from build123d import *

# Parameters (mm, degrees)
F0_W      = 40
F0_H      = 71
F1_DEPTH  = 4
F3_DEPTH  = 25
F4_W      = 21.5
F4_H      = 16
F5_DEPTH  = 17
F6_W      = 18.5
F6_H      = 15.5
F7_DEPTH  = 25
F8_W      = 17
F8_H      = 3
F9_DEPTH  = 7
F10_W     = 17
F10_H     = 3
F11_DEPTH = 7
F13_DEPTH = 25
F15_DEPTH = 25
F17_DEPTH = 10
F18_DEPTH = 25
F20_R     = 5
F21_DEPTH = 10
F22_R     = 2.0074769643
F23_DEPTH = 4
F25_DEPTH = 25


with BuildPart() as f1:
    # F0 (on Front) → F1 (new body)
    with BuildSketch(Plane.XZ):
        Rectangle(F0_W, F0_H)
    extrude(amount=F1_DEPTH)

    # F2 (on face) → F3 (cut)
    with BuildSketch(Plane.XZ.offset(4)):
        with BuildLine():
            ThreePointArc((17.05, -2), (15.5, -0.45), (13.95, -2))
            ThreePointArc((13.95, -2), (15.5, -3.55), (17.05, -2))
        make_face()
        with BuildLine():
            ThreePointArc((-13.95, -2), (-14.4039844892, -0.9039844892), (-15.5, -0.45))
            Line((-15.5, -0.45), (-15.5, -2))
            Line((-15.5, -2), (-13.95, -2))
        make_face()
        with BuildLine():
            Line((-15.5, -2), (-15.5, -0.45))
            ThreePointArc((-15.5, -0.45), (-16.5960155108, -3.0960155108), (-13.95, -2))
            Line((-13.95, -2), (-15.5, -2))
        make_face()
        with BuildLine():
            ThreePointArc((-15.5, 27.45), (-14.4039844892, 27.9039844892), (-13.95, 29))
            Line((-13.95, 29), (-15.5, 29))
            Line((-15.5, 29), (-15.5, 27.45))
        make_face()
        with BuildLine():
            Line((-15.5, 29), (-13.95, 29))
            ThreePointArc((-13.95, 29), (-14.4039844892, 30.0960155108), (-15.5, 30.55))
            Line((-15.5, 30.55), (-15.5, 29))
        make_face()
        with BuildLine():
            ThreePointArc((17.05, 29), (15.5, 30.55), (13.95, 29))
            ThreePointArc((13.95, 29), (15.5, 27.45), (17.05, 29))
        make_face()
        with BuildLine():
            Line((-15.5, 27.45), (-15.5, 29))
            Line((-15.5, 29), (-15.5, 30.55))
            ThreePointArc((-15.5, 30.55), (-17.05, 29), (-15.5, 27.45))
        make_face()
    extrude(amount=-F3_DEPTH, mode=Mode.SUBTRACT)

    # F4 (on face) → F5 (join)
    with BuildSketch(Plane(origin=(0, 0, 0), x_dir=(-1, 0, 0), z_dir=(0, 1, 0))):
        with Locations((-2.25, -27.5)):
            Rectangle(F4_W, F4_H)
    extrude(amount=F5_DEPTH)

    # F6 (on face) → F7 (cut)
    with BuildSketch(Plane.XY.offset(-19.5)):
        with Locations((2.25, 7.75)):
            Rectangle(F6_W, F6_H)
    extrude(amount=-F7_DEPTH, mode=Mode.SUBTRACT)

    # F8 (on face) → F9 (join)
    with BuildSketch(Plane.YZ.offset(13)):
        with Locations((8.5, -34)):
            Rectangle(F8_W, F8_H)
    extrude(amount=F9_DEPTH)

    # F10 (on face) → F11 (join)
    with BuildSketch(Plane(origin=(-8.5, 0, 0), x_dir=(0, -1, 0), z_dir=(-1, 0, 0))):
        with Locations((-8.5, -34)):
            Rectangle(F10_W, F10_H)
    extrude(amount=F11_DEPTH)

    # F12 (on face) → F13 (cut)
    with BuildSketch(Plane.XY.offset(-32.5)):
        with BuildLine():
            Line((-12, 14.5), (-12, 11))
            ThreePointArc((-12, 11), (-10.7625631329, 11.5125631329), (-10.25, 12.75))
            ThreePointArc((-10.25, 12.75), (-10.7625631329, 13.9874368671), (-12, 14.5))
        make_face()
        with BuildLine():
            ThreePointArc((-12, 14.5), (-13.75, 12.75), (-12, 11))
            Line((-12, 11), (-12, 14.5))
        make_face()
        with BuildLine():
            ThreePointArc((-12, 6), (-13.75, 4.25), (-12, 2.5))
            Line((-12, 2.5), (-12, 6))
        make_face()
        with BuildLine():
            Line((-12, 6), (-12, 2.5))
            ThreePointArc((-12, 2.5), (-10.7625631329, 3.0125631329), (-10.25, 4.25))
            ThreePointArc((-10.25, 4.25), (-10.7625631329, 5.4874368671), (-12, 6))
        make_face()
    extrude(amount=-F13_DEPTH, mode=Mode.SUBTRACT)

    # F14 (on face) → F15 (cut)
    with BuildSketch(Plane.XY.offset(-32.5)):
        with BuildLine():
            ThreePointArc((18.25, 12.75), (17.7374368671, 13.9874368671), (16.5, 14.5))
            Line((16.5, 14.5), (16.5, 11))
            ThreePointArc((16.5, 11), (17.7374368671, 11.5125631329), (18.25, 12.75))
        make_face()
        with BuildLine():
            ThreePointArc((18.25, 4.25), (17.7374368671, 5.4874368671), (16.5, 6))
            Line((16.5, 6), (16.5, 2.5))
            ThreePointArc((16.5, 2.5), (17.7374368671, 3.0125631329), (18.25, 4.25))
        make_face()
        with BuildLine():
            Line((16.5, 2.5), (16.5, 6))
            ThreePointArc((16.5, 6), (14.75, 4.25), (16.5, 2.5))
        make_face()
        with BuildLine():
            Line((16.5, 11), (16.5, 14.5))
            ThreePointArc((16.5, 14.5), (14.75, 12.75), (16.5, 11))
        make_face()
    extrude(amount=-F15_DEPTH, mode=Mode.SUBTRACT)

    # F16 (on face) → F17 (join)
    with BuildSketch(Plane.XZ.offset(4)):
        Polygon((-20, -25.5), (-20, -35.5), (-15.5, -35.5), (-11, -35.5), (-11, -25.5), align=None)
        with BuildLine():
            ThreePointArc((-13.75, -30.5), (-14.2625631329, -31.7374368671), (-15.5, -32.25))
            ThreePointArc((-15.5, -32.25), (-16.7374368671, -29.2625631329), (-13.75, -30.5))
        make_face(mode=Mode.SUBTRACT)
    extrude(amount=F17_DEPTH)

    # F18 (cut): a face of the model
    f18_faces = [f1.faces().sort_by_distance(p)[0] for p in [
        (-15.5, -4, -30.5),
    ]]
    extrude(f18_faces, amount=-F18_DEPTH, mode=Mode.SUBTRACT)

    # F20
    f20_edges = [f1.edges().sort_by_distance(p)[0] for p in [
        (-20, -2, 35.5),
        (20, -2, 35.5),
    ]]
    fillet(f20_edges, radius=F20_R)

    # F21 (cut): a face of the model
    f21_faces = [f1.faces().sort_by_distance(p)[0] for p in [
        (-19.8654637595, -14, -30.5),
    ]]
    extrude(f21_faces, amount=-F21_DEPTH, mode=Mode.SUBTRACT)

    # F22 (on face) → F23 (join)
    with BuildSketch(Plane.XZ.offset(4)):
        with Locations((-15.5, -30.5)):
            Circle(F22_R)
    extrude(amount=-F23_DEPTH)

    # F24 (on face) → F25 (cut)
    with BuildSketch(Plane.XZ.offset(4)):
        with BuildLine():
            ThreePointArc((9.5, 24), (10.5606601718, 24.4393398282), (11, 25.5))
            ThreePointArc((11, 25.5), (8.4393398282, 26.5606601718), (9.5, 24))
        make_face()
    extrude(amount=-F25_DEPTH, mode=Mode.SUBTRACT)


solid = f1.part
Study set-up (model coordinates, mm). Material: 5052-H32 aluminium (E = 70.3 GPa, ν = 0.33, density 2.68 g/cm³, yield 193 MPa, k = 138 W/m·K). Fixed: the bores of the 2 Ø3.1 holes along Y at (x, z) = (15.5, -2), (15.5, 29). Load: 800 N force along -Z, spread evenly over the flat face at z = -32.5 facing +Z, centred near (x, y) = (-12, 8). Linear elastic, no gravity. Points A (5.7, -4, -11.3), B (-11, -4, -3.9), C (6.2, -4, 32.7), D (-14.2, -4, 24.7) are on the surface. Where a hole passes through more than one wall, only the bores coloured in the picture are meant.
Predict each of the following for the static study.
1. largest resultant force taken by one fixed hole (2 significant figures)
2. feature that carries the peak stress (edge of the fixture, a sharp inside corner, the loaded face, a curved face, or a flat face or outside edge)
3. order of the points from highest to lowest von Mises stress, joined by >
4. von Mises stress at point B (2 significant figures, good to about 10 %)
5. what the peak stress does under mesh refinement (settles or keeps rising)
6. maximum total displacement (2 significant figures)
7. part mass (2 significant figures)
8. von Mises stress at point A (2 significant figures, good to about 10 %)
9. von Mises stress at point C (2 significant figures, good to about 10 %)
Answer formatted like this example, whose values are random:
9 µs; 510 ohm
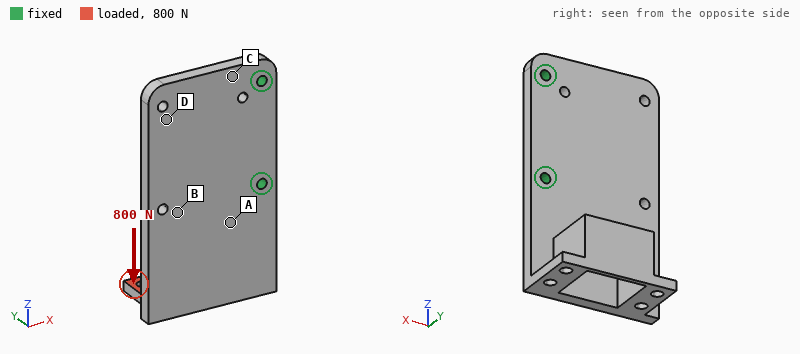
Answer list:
810 N; edge of the fixture; A > B > C > D; 54 MPa; keeps rising; 0.65 mm; 35 g; 73 MPa; 26 MPa
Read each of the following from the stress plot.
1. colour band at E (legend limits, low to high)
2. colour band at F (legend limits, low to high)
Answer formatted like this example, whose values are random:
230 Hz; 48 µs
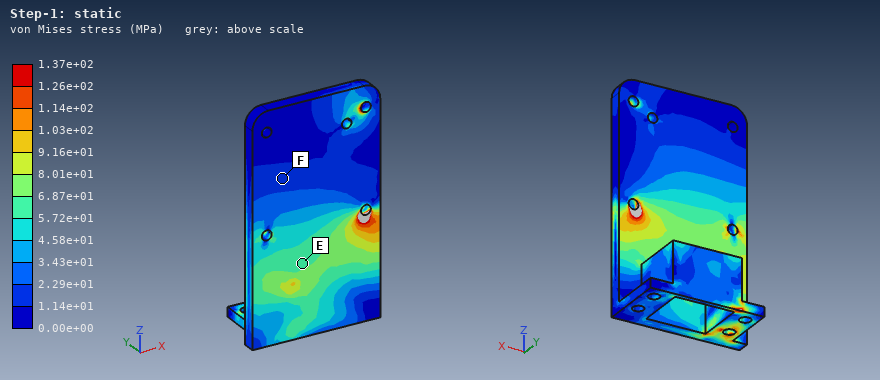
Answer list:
5.72e+01 to 6.87e+01 MPa; 1.14e+01 to 2.29e+01 MPa
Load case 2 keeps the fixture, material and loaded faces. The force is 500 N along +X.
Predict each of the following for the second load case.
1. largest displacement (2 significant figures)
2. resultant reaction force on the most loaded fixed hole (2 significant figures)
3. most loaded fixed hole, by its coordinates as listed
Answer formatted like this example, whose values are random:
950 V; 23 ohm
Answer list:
0.34 mm; 980 N; (15.5, -2)
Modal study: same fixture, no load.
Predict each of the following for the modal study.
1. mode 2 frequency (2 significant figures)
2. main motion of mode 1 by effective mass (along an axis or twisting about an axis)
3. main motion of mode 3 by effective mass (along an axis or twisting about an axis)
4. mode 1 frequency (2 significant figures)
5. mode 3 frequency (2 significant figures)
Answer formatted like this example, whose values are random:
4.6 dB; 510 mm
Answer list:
2100 Hz; along Y; along Y; 1300 Hz; 3400 Hz
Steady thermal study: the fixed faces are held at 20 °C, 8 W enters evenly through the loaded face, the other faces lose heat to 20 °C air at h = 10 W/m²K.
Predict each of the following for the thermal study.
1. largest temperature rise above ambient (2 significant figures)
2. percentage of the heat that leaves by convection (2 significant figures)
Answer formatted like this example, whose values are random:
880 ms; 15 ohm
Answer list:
31 K; 9.9 %
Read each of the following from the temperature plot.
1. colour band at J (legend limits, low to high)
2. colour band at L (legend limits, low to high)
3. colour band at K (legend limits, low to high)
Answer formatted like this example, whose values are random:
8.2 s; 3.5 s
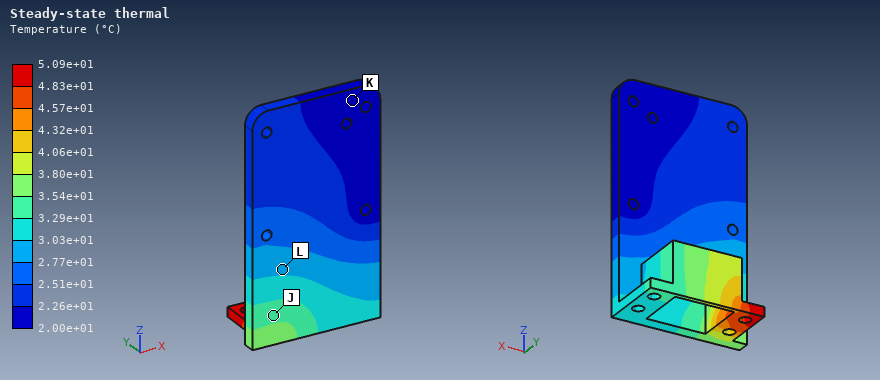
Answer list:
3.29e+01 to 3.54e+01 °C; 2.77e+01 to 3.03e+01 °C; 2.00e+01 to 2.26e+01 °C
